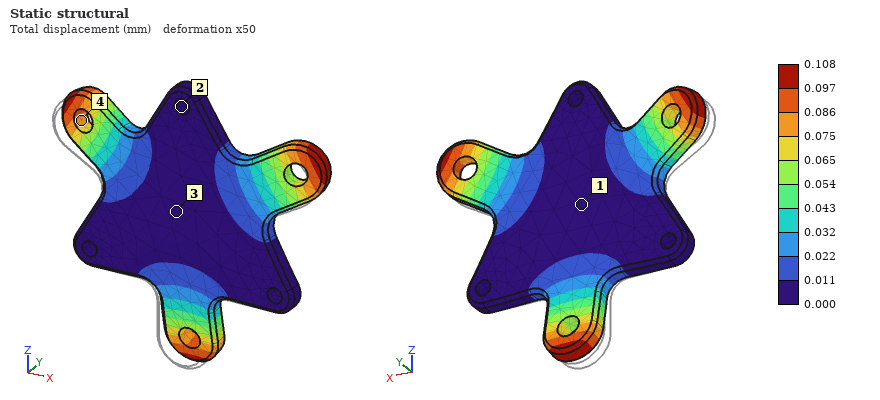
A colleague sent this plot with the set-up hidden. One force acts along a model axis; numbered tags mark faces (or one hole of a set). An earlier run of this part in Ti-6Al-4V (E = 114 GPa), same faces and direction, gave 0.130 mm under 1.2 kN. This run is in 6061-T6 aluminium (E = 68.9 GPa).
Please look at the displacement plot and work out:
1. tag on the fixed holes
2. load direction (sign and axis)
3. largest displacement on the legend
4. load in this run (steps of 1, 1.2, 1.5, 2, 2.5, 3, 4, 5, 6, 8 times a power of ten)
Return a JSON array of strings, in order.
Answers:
["2", "+Y", "0.108 mm", "600 N"]
